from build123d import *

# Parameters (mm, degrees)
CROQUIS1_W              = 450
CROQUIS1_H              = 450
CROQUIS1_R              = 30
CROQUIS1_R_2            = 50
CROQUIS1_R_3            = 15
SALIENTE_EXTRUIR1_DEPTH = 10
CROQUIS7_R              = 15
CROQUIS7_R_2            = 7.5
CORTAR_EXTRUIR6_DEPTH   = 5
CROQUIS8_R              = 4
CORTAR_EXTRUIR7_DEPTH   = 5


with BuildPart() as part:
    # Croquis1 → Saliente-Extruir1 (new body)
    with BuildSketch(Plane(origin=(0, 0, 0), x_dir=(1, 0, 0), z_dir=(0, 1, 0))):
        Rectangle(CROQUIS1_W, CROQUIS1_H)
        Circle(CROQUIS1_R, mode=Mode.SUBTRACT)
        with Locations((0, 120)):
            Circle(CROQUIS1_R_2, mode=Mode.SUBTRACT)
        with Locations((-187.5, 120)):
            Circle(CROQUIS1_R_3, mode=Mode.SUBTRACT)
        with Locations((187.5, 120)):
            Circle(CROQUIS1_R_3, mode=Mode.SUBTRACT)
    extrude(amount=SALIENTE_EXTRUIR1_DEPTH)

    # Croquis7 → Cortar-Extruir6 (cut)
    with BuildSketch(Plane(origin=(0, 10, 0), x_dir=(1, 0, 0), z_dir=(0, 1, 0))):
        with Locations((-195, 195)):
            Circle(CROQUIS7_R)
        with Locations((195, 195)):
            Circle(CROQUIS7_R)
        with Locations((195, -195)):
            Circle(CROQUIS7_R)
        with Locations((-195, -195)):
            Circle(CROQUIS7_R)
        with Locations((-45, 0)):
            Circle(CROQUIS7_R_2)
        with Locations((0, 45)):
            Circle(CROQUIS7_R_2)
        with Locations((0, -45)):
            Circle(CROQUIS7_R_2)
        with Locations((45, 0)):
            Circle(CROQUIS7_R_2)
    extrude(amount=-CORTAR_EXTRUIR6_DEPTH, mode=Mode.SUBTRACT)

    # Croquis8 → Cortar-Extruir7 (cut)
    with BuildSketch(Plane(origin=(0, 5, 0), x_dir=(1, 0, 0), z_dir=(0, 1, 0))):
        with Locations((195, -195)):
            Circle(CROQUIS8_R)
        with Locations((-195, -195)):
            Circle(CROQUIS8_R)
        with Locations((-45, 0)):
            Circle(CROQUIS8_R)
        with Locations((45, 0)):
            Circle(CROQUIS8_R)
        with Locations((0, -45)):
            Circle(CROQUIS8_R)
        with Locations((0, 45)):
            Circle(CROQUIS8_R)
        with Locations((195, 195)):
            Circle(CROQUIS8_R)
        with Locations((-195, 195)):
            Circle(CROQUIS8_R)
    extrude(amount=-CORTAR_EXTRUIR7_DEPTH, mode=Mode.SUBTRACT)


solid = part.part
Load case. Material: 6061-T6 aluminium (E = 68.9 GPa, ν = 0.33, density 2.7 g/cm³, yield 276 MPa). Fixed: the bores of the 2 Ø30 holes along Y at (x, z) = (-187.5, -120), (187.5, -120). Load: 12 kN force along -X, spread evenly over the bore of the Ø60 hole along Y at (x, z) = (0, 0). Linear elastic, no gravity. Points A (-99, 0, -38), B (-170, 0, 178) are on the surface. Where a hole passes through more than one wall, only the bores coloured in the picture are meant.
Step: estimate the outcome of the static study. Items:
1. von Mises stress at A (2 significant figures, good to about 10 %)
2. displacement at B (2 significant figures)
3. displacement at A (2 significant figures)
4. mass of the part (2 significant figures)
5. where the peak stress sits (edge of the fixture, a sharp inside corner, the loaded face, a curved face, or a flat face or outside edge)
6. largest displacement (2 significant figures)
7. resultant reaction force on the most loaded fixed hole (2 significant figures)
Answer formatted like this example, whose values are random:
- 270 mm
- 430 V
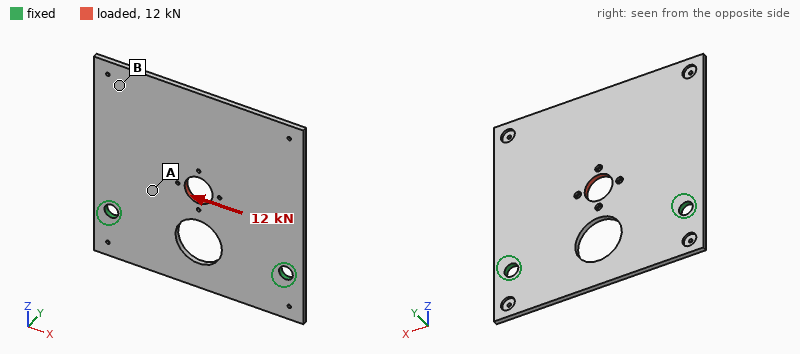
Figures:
- 5.6 MPa
- 27 µm
- 17 µm
- 5.1 kg
- a curved face
- 30 µm
- 7.0 kN
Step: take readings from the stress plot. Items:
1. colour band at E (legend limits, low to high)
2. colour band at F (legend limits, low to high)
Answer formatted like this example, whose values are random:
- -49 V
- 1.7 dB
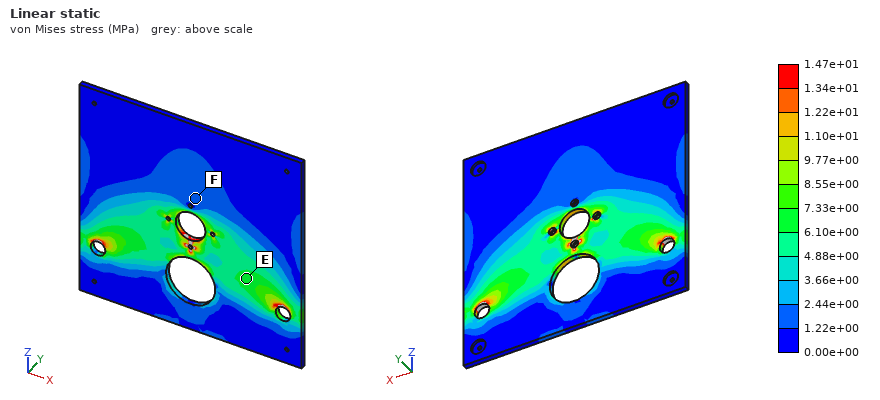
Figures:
- 6.10e+00 to 7.33e+00 MPa
- 1.22e+00 to 2.44e+00 MPa
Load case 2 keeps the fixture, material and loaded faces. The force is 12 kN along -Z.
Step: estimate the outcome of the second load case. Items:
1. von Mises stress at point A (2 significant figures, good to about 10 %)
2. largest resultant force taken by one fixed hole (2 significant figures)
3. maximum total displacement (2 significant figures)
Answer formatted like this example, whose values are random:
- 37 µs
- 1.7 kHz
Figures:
- 3.2 MPa
- 6.3 kN
- 27 µm
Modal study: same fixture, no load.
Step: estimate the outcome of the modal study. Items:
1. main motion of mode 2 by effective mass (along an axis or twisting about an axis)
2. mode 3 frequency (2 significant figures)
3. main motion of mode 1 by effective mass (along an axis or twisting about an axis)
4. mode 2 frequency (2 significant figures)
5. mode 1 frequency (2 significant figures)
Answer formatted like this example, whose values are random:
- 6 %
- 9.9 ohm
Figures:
- twisting about Z
- 320 Hz
- along Y
- 140 Hz
- 61 Hz
